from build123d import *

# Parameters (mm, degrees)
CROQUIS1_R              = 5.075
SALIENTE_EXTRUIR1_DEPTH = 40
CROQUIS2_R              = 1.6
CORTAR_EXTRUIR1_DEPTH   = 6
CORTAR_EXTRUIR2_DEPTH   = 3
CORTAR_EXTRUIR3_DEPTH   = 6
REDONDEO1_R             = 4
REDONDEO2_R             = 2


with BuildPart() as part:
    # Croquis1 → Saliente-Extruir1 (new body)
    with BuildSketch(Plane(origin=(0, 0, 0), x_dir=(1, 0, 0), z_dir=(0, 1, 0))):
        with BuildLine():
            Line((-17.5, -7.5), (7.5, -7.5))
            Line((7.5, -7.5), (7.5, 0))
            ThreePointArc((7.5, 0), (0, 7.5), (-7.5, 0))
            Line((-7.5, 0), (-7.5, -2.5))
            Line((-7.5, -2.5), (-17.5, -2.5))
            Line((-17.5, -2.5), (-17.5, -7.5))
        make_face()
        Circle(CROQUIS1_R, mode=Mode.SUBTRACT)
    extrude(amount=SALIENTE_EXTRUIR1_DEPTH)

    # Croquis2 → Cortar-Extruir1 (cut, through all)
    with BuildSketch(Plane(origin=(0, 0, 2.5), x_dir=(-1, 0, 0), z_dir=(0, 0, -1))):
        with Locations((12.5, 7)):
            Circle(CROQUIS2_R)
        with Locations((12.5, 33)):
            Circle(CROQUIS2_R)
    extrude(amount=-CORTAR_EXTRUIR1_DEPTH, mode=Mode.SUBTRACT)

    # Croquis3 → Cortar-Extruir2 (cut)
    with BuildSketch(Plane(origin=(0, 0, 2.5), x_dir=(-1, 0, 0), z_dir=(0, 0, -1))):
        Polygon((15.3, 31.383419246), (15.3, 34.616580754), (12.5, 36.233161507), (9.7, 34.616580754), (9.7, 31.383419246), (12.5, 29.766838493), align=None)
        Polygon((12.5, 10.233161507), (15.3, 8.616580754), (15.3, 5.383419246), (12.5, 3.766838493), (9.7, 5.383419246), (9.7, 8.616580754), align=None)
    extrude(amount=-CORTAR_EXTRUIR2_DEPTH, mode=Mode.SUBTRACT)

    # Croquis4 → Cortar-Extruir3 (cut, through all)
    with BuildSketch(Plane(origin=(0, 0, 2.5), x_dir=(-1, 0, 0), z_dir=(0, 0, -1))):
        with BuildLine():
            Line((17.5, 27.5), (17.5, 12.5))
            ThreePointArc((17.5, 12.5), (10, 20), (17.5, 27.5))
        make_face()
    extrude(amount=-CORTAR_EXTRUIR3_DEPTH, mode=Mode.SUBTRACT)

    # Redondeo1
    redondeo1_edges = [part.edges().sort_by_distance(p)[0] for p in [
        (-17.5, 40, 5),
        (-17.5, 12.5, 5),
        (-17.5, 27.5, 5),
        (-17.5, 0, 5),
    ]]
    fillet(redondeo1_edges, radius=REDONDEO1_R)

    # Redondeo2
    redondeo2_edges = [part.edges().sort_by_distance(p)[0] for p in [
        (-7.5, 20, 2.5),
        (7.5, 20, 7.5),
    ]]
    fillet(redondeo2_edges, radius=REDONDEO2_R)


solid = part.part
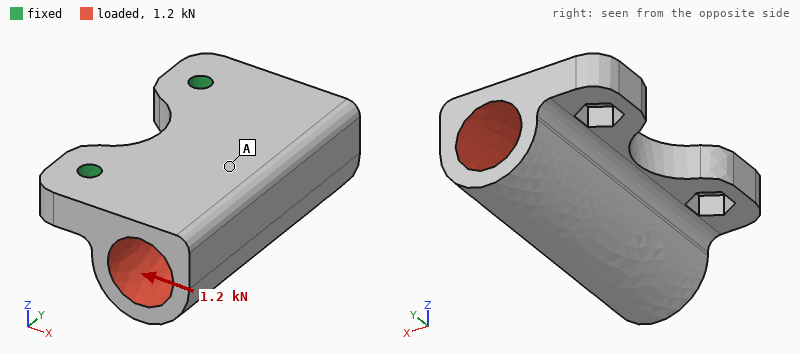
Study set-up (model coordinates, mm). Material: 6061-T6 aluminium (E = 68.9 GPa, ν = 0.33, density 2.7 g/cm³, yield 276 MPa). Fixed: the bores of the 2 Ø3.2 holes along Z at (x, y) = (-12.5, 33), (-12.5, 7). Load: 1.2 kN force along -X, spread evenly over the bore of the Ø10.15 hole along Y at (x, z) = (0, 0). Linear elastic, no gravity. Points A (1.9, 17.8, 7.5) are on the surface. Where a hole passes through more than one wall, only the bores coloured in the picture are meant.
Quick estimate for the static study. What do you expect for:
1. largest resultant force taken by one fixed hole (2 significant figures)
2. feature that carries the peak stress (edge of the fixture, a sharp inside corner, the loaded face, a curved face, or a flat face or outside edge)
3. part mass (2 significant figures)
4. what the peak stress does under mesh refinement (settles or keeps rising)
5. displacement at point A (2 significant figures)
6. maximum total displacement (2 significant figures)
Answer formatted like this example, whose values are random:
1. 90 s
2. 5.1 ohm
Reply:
1. 620 N
2. edge of the fixture
3. 16 g
4. keeps rising
5. 0.088 mm
6. 0.15 mm
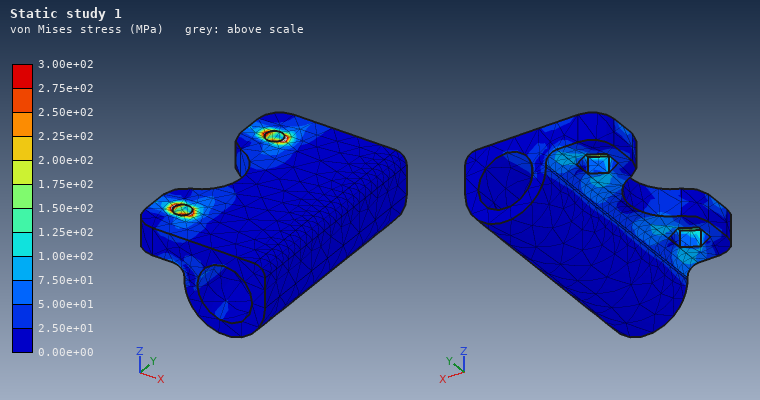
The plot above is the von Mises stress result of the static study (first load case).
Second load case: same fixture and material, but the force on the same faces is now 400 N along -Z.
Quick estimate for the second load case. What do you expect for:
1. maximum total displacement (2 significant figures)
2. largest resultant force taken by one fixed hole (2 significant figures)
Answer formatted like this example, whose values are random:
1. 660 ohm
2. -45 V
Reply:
1. 85 µm
2. 200 N
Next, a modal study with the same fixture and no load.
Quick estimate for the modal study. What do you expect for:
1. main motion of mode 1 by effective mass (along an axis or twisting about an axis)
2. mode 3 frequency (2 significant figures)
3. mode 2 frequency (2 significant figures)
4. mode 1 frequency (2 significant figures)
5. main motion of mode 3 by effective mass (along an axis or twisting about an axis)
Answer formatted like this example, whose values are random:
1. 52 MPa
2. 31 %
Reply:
1. along Z
2. 16 kHz
3. 13 kHz
4. 3300 Hz
5. along Y
